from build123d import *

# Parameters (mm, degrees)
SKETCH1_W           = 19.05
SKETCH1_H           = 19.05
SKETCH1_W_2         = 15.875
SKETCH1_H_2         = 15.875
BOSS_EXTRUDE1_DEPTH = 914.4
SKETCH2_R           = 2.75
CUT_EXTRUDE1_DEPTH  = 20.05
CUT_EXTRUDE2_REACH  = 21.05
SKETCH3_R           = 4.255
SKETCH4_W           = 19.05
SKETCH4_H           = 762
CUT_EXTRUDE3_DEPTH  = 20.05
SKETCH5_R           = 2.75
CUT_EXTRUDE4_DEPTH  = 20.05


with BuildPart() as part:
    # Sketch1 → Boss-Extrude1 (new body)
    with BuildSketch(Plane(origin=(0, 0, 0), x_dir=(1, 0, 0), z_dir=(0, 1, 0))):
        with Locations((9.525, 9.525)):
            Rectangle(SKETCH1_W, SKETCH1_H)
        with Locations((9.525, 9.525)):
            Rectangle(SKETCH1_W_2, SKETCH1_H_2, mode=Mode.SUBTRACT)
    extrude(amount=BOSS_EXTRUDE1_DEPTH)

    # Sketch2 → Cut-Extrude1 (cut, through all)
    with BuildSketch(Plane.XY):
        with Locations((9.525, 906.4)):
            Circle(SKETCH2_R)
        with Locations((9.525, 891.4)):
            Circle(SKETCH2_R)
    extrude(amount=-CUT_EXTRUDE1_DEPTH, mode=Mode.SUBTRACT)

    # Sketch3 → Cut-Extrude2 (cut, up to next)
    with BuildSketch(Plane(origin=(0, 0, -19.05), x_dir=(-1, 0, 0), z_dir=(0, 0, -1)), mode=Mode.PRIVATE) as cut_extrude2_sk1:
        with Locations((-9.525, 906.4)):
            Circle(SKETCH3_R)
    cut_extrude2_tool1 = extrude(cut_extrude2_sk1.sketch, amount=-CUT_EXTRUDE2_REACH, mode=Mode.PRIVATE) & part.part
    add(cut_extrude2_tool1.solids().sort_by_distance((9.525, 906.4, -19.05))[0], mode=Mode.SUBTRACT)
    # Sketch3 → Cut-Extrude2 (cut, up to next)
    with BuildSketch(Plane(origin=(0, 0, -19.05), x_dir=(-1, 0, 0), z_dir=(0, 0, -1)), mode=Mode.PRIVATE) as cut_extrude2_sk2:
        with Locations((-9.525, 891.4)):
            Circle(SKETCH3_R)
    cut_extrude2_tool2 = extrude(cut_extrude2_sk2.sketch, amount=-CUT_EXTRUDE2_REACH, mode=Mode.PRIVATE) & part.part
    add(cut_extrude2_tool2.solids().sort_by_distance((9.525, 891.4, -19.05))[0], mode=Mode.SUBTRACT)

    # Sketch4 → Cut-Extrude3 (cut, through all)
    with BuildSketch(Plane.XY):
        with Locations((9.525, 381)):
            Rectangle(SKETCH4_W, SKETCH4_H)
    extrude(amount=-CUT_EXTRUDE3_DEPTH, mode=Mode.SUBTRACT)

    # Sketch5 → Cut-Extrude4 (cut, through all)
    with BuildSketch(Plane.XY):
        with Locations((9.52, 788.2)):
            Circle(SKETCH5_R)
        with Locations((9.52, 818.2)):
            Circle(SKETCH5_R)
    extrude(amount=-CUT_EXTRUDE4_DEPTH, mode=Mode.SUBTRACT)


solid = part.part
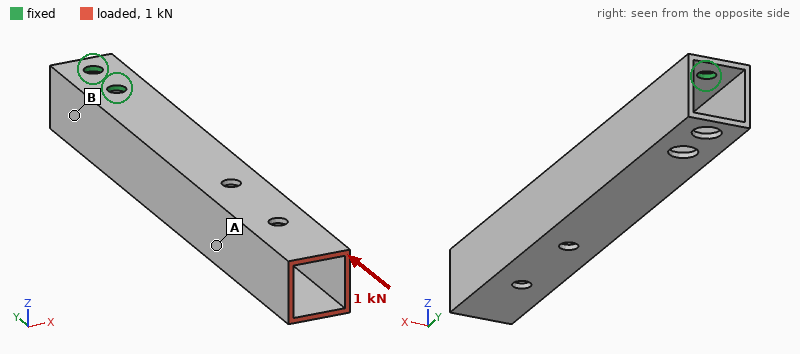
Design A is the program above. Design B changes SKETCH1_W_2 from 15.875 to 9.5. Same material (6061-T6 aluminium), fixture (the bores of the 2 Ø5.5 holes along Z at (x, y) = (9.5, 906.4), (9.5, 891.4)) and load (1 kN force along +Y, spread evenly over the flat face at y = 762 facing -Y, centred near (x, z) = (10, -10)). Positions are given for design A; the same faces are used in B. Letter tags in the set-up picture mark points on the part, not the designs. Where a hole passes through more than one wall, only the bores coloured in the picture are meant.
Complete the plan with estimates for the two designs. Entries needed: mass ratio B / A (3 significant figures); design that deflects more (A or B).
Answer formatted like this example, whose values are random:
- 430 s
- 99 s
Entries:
- 1.94
- A
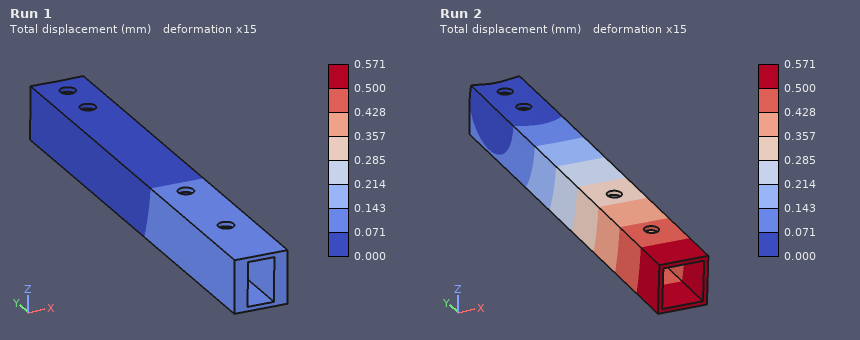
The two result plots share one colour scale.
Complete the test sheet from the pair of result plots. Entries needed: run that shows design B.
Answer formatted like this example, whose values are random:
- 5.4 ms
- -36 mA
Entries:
- Run 1
